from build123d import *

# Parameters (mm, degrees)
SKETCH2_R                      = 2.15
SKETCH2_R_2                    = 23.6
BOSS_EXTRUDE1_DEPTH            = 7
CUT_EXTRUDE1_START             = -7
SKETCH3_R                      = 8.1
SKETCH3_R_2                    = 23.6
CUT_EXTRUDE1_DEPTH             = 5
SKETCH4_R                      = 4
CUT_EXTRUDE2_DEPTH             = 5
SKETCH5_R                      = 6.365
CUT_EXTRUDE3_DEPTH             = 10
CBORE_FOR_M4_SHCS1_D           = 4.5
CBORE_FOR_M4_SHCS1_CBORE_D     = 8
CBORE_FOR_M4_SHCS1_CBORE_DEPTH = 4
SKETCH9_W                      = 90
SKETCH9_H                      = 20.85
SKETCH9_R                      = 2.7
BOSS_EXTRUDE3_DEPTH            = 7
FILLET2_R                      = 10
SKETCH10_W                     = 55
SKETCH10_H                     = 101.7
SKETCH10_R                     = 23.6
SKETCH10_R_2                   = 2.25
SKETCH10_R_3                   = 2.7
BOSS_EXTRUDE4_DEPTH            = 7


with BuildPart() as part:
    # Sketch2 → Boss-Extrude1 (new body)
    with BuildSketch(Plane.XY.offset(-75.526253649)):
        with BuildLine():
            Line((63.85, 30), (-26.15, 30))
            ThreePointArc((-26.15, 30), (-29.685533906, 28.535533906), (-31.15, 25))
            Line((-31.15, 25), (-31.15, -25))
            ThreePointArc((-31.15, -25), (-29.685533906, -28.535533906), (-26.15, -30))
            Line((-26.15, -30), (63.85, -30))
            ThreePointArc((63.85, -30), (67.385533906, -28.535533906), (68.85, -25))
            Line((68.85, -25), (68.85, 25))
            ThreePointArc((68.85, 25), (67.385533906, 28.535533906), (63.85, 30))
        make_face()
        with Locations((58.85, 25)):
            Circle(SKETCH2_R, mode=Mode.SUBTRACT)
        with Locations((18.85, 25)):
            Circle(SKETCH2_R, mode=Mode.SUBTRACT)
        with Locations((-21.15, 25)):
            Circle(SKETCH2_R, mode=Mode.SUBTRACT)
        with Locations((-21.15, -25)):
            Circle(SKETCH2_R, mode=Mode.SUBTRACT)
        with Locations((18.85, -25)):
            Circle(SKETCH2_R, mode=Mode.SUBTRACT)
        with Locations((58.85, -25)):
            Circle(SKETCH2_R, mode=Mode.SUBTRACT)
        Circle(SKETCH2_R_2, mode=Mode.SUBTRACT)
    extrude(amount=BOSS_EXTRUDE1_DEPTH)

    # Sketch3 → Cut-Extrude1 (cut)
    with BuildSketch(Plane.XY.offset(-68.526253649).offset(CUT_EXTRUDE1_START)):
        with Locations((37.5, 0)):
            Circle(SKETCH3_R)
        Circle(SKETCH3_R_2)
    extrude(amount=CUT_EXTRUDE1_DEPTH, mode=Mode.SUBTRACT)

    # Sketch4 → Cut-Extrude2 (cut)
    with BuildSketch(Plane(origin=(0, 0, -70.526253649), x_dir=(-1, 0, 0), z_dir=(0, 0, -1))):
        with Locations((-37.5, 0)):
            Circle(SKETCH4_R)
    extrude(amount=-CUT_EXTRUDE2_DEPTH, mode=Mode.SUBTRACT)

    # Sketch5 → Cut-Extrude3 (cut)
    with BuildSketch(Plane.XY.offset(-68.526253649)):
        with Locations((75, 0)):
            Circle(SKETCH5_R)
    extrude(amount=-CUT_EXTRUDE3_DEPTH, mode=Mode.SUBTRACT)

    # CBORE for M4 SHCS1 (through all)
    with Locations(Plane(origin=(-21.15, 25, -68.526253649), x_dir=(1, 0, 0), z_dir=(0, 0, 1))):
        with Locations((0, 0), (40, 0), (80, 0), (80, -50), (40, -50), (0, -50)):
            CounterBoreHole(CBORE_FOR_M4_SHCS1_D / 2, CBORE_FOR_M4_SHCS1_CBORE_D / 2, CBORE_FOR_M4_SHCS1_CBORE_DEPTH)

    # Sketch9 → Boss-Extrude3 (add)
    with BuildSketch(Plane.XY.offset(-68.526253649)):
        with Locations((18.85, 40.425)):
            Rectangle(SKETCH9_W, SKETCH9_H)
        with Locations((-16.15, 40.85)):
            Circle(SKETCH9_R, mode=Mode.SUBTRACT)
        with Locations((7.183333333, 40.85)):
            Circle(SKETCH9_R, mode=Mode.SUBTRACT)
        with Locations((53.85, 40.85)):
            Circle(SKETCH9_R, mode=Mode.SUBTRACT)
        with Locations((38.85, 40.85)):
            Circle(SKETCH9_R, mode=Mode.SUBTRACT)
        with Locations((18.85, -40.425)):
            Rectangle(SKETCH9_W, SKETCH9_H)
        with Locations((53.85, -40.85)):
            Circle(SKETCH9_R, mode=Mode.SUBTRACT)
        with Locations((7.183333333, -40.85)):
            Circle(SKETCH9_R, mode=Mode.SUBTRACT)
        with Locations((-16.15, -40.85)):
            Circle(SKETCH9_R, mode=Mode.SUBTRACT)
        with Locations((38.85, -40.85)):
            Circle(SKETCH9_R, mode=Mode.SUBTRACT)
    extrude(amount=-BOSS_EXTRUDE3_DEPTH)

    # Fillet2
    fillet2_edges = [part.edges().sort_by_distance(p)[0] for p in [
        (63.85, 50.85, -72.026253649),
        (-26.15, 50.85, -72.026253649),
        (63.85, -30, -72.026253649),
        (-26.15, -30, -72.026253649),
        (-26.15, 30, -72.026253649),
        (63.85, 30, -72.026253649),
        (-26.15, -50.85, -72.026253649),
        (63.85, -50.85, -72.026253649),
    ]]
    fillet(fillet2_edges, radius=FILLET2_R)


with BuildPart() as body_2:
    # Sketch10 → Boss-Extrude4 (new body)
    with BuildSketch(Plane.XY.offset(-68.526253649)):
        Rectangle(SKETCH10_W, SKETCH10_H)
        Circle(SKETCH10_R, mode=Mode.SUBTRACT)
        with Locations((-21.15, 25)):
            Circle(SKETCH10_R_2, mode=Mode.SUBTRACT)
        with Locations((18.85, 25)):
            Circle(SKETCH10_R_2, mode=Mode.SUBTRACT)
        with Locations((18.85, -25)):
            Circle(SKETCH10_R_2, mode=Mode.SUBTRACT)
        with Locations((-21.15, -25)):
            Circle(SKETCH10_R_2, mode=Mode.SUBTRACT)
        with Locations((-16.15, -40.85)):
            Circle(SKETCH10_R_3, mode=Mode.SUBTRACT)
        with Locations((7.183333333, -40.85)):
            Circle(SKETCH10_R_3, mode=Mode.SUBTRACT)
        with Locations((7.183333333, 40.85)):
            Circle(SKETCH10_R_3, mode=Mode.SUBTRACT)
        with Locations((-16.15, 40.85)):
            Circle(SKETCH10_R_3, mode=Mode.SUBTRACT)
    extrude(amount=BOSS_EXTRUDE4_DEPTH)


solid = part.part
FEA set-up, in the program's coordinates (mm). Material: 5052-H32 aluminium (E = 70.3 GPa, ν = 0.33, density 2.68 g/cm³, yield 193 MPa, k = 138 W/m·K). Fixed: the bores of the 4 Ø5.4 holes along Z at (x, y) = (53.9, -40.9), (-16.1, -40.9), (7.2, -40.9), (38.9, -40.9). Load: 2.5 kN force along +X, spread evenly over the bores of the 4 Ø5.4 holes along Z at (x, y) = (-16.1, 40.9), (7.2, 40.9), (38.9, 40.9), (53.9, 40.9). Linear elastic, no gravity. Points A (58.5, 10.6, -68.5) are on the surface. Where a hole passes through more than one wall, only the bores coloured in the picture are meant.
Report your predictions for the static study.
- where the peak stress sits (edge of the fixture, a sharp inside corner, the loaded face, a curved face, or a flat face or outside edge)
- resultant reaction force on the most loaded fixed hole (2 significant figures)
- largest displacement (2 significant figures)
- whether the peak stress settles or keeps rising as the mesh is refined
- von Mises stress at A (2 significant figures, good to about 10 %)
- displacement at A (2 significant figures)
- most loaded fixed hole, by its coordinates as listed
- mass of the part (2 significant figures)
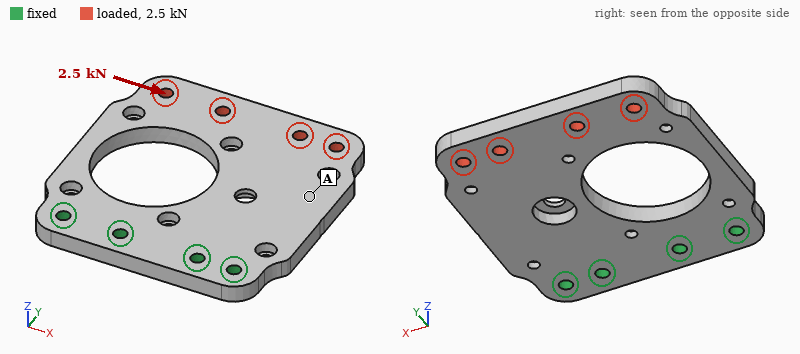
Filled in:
edge of the fixture
3.5 kN
90 µm
keeps rising
8.3 MPa
48 µm
(53.9, -40.9)
140 g
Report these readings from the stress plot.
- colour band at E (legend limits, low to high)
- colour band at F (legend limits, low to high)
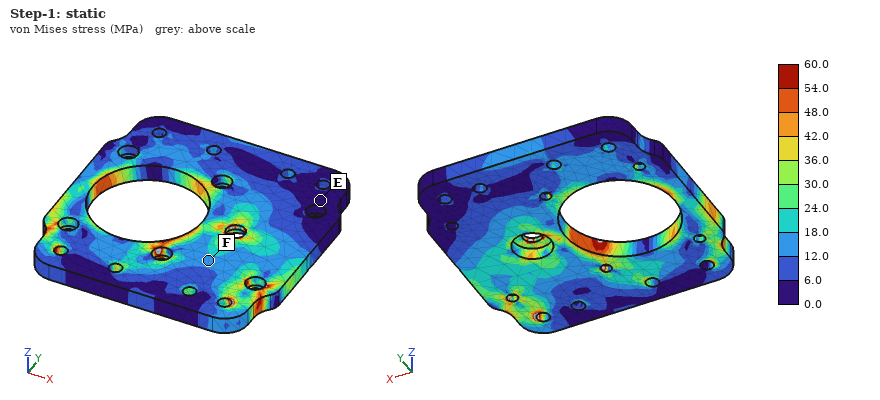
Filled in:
0.0 to 6.0 MPa
12.0 to 18.0 MPa
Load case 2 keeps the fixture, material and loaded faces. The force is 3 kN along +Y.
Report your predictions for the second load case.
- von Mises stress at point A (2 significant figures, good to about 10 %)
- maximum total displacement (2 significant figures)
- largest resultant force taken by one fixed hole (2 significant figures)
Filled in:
3.0 MPa
23 µm
1.0 kN
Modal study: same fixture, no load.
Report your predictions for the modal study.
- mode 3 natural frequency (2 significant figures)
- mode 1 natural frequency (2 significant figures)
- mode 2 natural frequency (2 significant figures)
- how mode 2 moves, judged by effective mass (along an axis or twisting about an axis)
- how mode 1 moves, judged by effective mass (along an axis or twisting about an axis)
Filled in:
3700 Hz
600 Hz
1400 Hz
twisting about Y
along Z
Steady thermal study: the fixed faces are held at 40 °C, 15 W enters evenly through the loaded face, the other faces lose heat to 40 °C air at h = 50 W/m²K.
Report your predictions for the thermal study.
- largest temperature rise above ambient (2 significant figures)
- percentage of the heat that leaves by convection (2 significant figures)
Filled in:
16 K
47 %
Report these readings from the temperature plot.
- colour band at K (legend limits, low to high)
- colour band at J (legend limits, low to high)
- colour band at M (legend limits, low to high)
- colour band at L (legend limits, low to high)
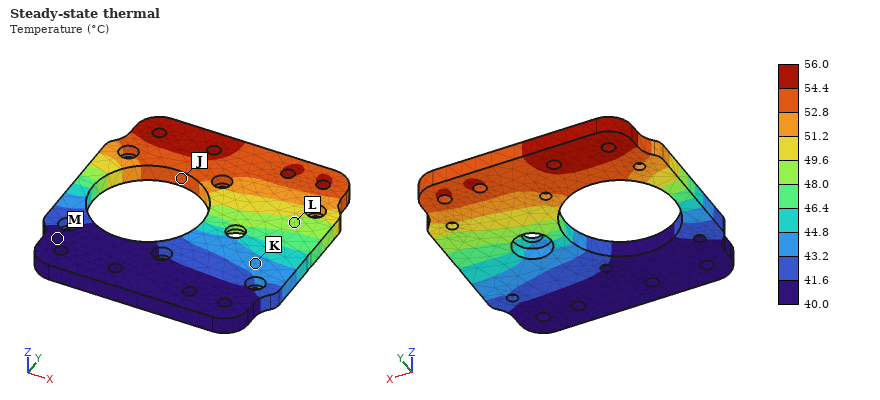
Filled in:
43.2 to 44.8 °C
52.8 to 54.4 °C
40.0 to 41.6 °C
48.0 to 49.6 °C
